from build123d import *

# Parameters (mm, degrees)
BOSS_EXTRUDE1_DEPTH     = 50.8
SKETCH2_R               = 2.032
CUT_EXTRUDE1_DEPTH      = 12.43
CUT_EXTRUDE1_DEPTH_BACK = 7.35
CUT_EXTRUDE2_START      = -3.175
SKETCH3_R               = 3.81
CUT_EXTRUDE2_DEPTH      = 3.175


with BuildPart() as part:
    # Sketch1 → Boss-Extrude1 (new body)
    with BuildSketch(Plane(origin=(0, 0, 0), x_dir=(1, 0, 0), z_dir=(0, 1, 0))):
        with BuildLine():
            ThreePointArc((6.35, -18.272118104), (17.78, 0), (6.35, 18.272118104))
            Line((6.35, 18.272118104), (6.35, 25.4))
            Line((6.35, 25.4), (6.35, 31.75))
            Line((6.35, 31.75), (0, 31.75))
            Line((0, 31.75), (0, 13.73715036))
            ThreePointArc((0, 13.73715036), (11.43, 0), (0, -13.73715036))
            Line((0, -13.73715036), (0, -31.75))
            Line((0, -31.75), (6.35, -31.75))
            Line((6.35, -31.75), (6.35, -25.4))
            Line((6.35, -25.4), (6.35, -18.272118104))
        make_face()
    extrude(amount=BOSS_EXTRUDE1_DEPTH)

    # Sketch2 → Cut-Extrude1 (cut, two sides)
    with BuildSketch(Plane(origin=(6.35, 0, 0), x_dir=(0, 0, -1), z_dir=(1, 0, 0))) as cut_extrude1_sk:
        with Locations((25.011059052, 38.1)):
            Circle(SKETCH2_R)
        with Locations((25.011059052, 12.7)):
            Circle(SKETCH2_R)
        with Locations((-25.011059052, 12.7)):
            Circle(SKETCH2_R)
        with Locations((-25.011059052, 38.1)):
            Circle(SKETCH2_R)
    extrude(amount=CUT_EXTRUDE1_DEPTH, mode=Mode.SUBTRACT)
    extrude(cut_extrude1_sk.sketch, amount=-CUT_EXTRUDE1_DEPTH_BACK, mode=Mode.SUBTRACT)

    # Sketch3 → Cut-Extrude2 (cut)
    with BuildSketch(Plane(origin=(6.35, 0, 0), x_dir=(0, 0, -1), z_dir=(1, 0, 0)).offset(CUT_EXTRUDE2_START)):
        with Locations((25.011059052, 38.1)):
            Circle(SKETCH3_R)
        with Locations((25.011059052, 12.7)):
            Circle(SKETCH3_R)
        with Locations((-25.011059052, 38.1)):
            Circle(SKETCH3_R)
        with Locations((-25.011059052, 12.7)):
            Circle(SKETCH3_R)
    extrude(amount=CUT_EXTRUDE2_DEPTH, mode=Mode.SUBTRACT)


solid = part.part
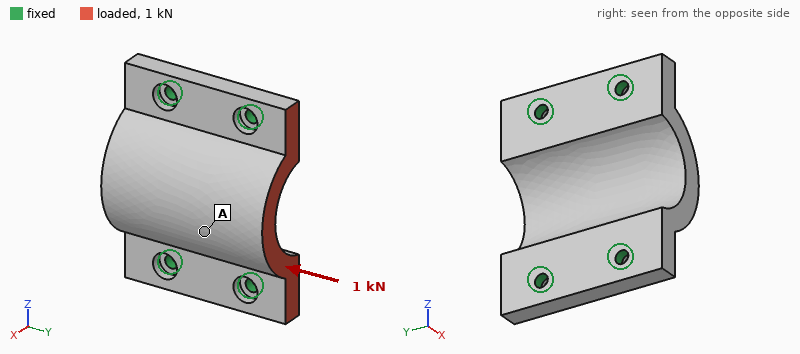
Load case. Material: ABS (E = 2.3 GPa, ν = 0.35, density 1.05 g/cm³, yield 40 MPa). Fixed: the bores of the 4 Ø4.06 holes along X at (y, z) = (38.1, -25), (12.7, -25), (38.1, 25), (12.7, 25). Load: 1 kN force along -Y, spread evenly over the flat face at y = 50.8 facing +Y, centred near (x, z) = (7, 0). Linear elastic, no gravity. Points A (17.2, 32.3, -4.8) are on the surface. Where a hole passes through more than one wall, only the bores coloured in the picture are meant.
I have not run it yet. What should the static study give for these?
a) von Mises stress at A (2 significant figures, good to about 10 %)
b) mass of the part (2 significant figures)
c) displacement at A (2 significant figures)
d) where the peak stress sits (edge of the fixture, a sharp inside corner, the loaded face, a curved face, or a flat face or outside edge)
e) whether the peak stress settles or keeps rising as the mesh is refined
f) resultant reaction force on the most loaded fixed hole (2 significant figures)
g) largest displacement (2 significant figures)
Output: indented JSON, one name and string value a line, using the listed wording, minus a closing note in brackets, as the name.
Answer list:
{
  "von Mises stress at A": "2.3 MPa",
  "mass of the part": "24 g",
  "displacement at A": "0.089 mm",
  "where the peak stress sits": "edge of the fixture",
  "whether the peak stress settles or keeps rising as the mesh is refined": "keeps rising",
  "resultant reaction force on the most loaded fixed hole": "370 N",
  "largest displacement": "0.15 mm"
}
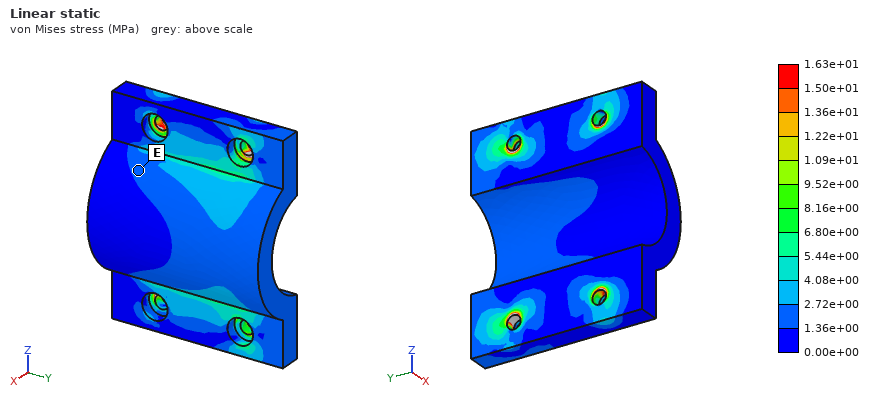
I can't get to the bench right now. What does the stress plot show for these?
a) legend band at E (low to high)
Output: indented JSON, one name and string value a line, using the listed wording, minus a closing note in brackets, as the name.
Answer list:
{
  "legend band at E": "1.36e+00 to 2.72e+00 MPa"
}
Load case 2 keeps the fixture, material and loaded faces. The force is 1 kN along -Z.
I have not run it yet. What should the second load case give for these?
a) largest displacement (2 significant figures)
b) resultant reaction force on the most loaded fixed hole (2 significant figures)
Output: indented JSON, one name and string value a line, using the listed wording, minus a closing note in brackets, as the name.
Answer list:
{
  "largest displacement": "0.21 mm",
  "resultant reaction force on the most loaded fixed hole": "500 N"
}
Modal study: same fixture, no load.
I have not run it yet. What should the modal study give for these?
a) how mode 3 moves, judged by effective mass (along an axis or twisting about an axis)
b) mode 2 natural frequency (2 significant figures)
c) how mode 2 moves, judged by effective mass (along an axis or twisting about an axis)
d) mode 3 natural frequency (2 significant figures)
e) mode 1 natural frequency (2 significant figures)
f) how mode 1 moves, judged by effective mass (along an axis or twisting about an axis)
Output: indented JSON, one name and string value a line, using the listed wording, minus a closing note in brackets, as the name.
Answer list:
{
  "how mode 3 moves, judged by effective mass": "along Z",
  "mode 2 natural frequency": "4000 Hz",
  "how mode 2 moves, judged by effective mass": "along X",
  "mode 3 natural frequency": "4900 Hz",
  "mode 1 natural frequency": "3000 Hz",
  "how mode 1 moves, judged by effective mass": "along Y"
}
